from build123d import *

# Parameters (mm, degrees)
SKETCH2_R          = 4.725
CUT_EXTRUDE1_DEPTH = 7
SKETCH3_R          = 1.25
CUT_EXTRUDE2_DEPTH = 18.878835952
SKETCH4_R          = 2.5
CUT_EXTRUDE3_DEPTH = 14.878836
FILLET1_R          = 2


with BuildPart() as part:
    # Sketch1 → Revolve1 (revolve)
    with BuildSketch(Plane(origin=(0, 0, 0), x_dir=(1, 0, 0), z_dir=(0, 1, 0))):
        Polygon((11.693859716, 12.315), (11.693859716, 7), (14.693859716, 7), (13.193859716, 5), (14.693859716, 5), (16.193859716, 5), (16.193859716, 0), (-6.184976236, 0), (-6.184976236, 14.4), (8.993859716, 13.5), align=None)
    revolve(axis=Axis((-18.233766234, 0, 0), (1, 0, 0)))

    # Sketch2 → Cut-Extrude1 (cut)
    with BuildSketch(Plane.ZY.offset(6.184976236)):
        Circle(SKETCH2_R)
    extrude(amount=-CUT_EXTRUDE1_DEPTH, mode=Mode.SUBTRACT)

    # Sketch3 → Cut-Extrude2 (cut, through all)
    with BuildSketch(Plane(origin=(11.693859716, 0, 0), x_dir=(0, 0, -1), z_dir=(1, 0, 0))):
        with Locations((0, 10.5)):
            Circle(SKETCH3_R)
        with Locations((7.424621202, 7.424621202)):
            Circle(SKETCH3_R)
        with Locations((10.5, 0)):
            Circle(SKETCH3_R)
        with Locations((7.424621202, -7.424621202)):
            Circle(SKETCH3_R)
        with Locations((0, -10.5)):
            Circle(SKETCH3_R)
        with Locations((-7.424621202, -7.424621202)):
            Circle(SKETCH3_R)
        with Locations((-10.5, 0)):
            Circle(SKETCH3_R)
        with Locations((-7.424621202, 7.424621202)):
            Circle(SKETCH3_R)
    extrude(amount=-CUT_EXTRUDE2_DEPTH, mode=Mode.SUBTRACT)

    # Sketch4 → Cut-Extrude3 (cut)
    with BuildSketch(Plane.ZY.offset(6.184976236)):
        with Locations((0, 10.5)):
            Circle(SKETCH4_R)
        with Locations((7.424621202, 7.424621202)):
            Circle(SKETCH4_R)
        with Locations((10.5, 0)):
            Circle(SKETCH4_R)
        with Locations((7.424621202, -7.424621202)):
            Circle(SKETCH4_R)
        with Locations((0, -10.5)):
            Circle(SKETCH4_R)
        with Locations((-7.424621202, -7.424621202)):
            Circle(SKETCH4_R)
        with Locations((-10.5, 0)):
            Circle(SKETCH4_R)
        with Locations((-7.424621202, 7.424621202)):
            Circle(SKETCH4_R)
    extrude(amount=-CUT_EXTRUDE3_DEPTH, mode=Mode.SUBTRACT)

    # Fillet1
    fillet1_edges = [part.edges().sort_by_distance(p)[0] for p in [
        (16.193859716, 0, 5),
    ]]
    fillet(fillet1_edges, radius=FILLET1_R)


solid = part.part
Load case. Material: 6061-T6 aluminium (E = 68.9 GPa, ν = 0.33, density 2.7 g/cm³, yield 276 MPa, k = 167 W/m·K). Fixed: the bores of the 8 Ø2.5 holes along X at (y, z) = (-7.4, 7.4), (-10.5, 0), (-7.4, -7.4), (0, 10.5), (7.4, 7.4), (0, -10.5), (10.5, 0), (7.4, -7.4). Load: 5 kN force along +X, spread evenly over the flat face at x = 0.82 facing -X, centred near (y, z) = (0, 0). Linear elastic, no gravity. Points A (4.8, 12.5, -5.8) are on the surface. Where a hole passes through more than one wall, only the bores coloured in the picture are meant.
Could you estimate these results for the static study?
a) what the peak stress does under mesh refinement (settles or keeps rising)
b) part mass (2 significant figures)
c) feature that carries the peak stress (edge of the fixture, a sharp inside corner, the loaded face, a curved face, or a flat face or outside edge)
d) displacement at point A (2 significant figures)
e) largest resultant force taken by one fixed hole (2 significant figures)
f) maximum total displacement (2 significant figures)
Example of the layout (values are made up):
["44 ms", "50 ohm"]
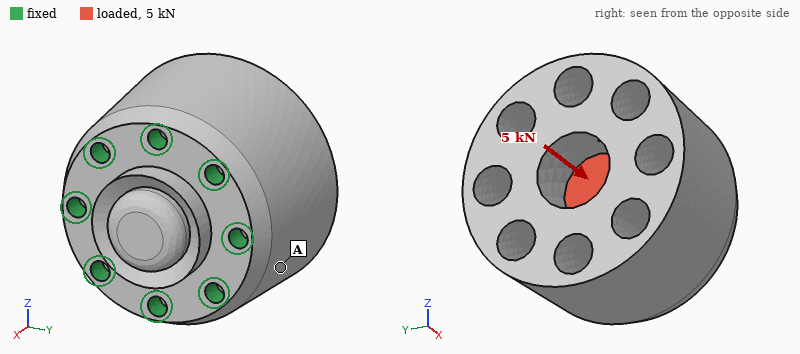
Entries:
["keeps rising", "22 g", "edge of the fixture", "1.8 µm", "660 N", "9.0 µm"]
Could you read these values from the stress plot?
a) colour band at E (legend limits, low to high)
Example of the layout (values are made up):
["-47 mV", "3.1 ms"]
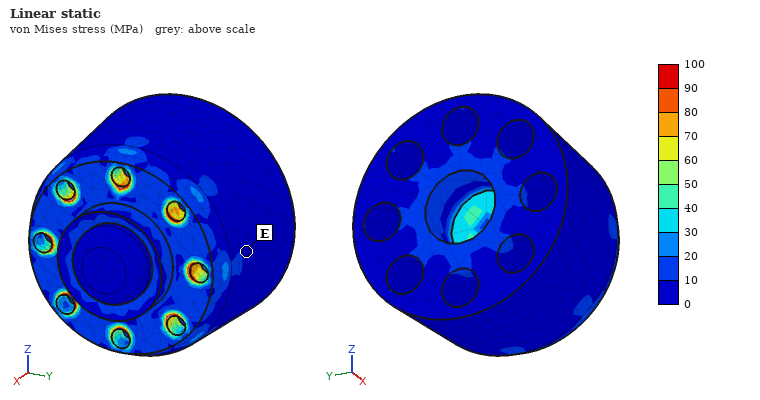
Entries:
["0 to 10 MPa"]
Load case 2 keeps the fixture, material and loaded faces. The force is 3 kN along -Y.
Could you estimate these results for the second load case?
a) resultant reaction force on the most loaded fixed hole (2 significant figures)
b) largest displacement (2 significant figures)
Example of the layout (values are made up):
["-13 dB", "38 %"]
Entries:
["820 N", "9.1 µm"]
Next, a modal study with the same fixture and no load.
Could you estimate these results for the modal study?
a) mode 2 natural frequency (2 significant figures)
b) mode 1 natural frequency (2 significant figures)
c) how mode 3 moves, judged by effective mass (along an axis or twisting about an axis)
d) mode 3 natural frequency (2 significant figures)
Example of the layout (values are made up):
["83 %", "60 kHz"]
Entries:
["27 kHz", "27 kHz", "twisting about X", "37 kHz"]
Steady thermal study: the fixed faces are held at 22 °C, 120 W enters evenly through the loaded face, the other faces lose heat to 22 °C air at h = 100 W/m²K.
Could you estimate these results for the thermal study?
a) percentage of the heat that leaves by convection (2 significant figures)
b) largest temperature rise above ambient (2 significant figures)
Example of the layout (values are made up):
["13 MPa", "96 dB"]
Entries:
["4.7 %", "47 K"]
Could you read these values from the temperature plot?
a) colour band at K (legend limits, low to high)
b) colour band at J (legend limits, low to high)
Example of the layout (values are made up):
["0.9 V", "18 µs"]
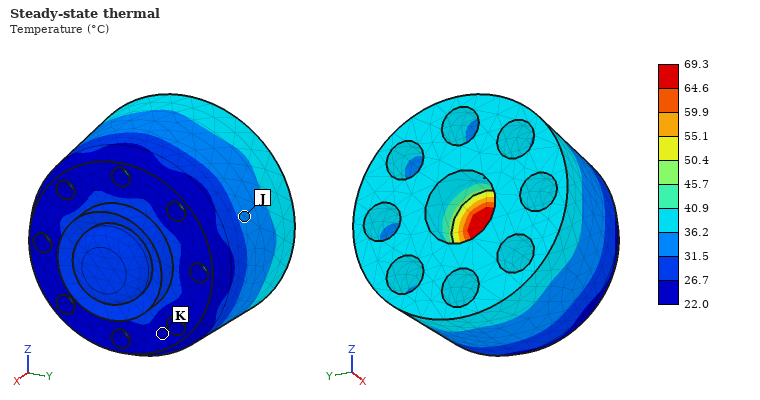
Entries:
["22.0 to 26.7 °C", "31.5 to 36.2 °C"]
